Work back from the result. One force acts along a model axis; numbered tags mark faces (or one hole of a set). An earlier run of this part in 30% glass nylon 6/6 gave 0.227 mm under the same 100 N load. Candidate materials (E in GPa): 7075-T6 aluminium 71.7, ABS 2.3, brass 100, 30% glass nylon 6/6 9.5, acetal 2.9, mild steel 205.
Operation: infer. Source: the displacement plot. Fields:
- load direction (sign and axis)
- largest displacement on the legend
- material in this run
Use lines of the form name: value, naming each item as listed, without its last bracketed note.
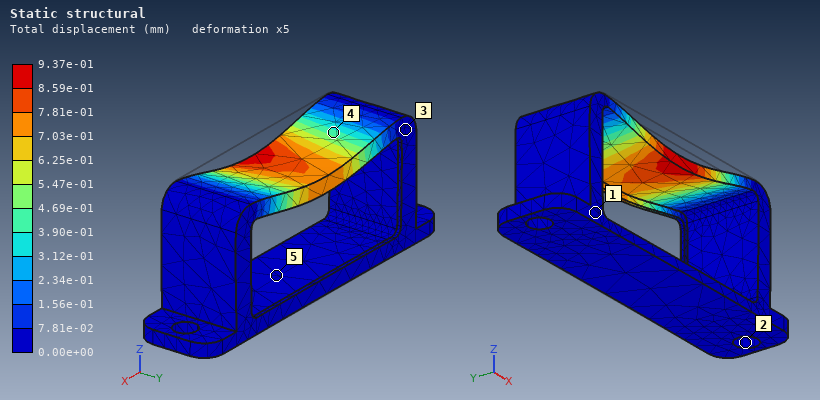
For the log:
load direction: -Z
largest displacement on the legend: 9.37e-01 mm
material in this run: ABS
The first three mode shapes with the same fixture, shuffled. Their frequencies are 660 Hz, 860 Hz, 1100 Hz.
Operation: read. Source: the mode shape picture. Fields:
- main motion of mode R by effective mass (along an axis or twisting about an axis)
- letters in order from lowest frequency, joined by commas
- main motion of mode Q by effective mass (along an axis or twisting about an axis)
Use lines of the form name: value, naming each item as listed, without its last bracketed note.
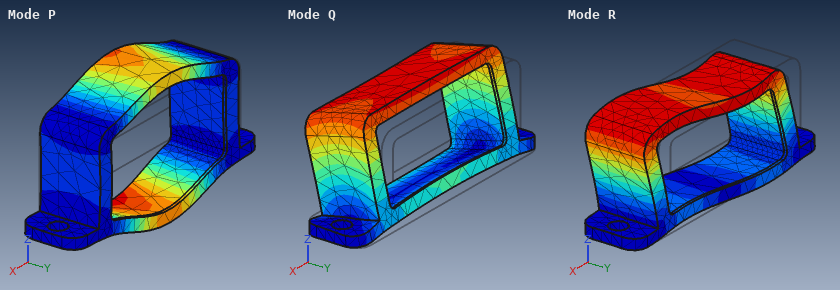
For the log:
main motion of mode R by effective mass: along X
letters in order from lowest frequency, joined by commas: R, Q, P
main motion of mode Q by effective mass: along Y
